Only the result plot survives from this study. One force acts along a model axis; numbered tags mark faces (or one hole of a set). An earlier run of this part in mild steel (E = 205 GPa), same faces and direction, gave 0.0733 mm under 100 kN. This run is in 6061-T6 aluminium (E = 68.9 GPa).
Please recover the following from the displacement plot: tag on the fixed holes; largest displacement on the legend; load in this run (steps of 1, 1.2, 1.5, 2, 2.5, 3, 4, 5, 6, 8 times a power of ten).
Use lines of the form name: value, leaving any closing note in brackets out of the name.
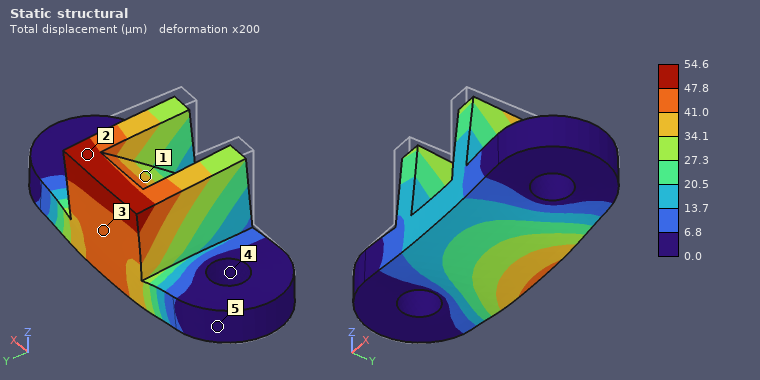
tag on the fixed holes: 4
largest displacement on the legend: 54.6 µm
load in this run: 25 kN
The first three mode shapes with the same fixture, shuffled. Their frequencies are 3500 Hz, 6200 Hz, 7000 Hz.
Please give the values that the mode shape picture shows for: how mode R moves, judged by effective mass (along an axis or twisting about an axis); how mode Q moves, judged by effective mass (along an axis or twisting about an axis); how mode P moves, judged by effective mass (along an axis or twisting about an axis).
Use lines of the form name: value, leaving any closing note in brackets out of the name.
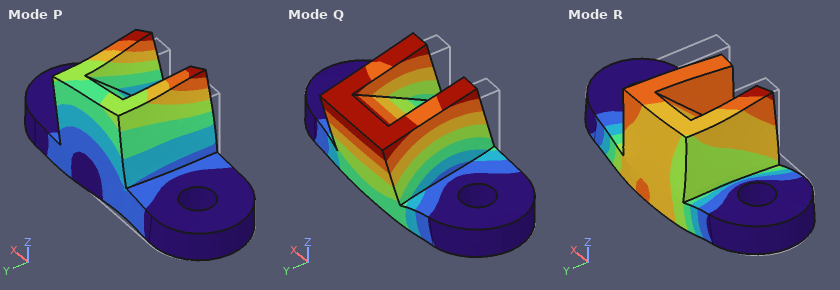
how mode R moves, judged by effective mass: along Z
how mode Q moves, judged by effective mass: along Y
how mode P moves, judged by effective mass: along X
